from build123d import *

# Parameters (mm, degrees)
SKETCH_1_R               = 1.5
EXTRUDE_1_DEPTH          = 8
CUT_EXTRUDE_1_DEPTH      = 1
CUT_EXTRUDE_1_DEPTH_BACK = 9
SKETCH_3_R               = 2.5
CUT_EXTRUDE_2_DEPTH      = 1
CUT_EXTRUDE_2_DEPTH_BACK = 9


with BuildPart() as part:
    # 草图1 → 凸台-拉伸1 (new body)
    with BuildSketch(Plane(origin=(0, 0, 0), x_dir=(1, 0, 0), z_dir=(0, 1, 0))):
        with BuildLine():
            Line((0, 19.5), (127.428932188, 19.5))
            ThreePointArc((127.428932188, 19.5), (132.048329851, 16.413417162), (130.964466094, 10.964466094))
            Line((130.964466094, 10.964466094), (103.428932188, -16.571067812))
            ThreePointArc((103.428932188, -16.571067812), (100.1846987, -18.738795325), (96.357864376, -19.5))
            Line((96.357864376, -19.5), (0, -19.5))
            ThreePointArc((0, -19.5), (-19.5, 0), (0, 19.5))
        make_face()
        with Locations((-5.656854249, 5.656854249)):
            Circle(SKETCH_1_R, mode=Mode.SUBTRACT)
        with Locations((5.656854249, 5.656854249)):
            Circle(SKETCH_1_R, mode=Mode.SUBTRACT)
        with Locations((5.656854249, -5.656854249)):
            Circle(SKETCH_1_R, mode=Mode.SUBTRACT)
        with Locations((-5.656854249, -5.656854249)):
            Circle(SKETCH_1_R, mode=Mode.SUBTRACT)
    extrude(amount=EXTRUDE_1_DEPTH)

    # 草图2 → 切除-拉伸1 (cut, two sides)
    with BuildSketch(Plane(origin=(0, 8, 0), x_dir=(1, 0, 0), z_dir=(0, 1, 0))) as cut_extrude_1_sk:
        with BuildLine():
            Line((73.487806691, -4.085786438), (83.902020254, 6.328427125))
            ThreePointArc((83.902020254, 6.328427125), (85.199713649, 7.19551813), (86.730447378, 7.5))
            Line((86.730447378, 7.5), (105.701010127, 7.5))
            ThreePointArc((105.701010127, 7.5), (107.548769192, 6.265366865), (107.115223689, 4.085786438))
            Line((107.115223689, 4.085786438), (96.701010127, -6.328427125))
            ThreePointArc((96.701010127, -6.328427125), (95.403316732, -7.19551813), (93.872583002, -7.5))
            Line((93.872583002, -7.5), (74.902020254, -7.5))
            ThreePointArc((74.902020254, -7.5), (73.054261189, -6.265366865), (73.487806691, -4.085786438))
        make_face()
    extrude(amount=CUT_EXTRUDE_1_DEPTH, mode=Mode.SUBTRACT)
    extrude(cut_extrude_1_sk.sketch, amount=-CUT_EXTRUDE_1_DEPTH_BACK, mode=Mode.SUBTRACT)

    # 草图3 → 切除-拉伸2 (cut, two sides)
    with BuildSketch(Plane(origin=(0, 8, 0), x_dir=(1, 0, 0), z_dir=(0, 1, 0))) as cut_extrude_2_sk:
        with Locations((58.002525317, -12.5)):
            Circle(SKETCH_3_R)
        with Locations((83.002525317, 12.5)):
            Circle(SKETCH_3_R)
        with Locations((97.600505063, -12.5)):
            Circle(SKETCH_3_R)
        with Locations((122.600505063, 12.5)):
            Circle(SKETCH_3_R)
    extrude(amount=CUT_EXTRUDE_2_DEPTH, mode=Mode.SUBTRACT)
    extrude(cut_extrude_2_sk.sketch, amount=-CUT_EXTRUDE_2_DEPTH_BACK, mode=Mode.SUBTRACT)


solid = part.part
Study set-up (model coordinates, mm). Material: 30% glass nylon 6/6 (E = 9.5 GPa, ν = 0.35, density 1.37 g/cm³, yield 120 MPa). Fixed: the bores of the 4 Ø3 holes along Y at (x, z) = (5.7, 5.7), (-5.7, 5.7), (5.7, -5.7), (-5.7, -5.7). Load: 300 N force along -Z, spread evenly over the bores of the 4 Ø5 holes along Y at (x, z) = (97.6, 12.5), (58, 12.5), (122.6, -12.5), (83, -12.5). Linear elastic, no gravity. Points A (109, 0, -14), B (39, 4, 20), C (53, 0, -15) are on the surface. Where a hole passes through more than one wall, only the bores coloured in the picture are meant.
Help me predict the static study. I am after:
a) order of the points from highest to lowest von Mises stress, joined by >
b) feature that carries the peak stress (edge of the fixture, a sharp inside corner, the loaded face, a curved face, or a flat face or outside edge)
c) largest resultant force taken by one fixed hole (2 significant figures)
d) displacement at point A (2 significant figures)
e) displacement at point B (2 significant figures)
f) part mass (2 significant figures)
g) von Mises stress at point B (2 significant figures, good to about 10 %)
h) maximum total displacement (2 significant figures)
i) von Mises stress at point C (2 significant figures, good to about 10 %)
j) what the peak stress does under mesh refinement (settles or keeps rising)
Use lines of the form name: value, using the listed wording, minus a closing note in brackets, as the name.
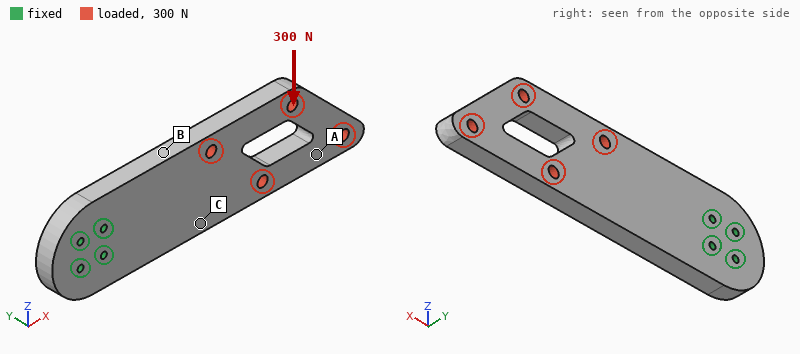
order of the points from highest to lowest von Mises stress, joined by >: B > C > A
feature that carries the peak stress: edge of the fixture
largest resultant force taken by one fixed hole: 970 N
displacement at point A: 0.39 mm
displacement at point B: 0.098 mm
part mass: 52 g
von Mises stress at point B: 7.7 MPa
maximum total displacement: 0.49 mm
von Mises stress at point C: 4.5 MPa
what the peak stress does under mesh refinement: keeps rising
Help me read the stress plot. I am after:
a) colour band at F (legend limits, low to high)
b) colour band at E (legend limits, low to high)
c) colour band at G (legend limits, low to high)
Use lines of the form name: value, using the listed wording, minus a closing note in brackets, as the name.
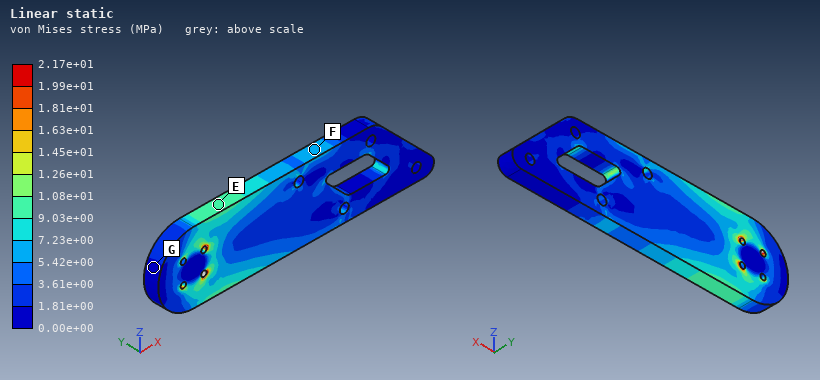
colour band at F: 5.42e+00 to 7.23e+00 MPa
colour band at E: 9.03e+00 to 1.08e+01 MPa
colour band at G: 0.00e+00 to 1.81e+00 MPa
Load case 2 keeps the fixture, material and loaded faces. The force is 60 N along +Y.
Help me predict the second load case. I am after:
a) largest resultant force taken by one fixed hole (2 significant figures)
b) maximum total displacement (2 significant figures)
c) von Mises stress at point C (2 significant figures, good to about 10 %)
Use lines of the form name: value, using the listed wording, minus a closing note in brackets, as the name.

largest resultant force taken by one fixed hole: 110 N
maximum total displacement: 1.5 mm
von Mises stress at point C: 5.7 MPa
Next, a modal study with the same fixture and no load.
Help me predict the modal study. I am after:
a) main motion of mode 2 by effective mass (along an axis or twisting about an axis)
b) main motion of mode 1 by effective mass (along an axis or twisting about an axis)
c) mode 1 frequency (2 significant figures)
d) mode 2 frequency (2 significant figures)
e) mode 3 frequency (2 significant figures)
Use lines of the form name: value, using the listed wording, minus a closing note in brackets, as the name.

main motion of mode 2 by effective mass: along Z
main motion of mode 1 by effective mass: along Y
mode 1 frequency: 280 Hz
mode 2 frequency: 1000 Hz
mode 3 frequency: 1300 Hz
